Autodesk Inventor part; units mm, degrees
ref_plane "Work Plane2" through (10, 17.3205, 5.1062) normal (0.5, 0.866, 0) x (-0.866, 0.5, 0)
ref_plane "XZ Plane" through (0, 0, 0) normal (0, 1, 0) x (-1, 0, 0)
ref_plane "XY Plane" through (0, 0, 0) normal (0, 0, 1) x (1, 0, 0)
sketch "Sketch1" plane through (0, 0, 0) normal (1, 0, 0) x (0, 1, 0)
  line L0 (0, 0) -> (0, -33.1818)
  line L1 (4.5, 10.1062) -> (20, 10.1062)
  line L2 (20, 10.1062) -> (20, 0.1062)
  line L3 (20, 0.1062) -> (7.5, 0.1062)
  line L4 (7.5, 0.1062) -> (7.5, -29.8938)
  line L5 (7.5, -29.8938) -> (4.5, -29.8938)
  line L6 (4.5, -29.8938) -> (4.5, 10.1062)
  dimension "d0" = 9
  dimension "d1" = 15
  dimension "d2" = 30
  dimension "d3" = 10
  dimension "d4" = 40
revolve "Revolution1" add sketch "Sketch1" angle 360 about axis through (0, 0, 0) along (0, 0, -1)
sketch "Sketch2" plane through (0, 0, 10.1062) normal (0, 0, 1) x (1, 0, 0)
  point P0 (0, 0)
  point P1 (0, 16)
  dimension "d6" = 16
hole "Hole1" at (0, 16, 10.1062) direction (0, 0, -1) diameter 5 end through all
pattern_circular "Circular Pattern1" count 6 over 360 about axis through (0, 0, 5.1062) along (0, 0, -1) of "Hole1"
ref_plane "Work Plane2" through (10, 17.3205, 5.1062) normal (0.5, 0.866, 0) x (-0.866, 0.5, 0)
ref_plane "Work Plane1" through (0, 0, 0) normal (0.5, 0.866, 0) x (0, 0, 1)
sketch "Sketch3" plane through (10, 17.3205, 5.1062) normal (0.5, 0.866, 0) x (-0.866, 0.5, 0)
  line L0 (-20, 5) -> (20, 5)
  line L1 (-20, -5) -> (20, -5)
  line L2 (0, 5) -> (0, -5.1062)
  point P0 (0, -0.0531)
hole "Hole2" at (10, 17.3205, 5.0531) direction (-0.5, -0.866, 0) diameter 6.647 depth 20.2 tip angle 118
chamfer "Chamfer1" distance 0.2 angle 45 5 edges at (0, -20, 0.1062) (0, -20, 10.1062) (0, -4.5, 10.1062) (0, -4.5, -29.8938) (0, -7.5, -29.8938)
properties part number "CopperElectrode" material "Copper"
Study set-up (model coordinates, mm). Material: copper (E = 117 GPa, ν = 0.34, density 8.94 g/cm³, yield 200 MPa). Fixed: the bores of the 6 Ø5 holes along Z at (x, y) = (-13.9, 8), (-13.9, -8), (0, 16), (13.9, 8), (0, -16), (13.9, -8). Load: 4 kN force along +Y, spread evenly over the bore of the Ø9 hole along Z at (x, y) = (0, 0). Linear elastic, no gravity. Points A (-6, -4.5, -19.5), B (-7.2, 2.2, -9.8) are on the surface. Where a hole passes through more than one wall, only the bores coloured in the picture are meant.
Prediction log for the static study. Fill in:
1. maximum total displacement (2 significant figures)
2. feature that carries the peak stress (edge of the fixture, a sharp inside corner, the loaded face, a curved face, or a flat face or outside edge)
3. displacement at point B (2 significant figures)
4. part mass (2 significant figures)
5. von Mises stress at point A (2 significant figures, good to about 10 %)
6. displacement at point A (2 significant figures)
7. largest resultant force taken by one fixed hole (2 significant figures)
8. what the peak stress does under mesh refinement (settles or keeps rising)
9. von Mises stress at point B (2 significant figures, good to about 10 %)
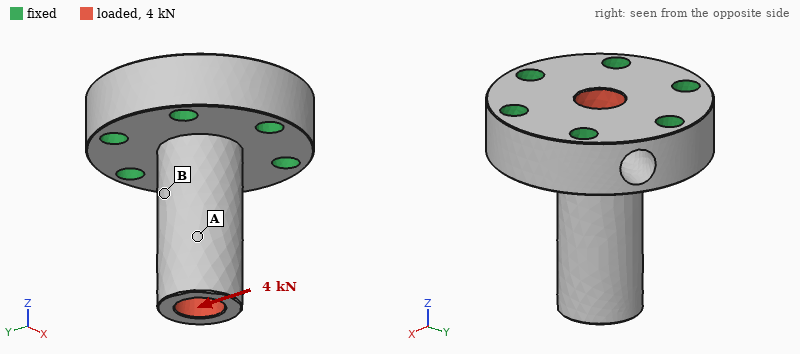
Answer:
88 µm
a sharp inside corner
26 µm
120 g
24 MPa
56 µm
2.0 kN
keeps rising
54 MPa
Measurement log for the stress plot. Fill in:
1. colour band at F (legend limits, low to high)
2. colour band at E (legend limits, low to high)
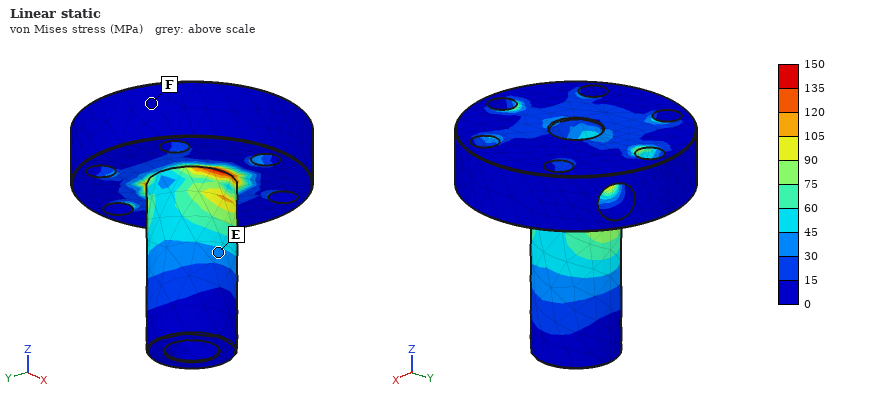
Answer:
0 to 15 MPa
30 to 45 MPa
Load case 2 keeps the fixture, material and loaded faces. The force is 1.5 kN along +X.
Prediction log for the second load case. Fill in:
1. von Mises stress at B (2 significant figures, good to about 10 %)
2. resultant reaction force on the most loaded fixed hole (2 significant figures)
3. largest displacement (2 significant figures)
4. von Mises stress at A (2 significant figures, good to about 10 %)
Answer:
25 MPa
680 N
32 µm
8.2 MPa
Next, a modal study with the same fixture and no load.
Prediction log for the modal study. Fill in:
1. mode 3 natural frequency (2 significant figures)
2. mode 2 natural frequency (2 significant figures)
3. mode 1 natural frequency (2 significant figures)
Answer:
17 kHz
6600 Hz
6500 Hz
